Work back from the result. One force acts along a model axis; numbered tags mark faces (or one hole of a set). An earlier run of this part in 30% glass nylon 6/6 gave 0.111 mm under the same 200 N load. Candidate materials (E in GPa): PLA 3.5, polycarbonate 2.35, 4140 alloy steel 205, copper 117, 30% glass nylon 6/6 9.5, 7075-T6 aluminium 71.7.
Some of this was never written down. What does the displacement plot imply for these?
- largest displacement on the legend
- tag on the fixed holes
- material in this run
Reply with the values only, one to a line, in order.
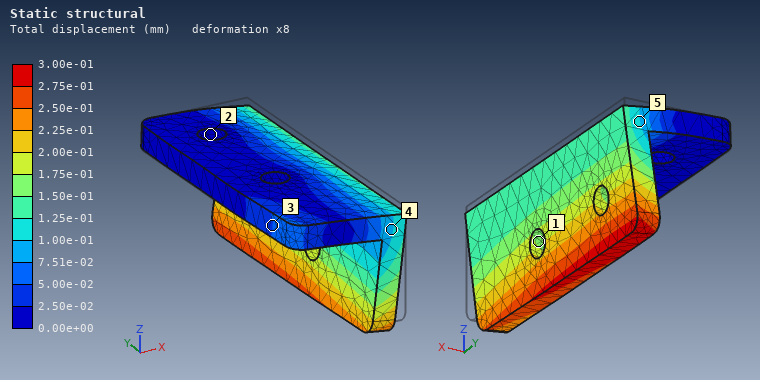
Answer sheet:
3.00e-01 mm
2
PLA
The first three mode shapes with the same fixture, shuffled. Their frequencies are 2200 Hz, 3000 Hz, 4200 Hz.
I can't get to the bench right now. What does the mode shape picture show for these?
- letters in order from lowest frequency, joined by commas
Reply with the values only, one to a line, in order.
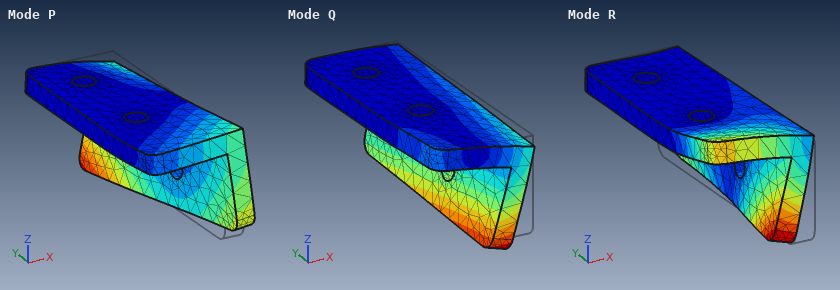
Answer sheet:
Q, P, R
